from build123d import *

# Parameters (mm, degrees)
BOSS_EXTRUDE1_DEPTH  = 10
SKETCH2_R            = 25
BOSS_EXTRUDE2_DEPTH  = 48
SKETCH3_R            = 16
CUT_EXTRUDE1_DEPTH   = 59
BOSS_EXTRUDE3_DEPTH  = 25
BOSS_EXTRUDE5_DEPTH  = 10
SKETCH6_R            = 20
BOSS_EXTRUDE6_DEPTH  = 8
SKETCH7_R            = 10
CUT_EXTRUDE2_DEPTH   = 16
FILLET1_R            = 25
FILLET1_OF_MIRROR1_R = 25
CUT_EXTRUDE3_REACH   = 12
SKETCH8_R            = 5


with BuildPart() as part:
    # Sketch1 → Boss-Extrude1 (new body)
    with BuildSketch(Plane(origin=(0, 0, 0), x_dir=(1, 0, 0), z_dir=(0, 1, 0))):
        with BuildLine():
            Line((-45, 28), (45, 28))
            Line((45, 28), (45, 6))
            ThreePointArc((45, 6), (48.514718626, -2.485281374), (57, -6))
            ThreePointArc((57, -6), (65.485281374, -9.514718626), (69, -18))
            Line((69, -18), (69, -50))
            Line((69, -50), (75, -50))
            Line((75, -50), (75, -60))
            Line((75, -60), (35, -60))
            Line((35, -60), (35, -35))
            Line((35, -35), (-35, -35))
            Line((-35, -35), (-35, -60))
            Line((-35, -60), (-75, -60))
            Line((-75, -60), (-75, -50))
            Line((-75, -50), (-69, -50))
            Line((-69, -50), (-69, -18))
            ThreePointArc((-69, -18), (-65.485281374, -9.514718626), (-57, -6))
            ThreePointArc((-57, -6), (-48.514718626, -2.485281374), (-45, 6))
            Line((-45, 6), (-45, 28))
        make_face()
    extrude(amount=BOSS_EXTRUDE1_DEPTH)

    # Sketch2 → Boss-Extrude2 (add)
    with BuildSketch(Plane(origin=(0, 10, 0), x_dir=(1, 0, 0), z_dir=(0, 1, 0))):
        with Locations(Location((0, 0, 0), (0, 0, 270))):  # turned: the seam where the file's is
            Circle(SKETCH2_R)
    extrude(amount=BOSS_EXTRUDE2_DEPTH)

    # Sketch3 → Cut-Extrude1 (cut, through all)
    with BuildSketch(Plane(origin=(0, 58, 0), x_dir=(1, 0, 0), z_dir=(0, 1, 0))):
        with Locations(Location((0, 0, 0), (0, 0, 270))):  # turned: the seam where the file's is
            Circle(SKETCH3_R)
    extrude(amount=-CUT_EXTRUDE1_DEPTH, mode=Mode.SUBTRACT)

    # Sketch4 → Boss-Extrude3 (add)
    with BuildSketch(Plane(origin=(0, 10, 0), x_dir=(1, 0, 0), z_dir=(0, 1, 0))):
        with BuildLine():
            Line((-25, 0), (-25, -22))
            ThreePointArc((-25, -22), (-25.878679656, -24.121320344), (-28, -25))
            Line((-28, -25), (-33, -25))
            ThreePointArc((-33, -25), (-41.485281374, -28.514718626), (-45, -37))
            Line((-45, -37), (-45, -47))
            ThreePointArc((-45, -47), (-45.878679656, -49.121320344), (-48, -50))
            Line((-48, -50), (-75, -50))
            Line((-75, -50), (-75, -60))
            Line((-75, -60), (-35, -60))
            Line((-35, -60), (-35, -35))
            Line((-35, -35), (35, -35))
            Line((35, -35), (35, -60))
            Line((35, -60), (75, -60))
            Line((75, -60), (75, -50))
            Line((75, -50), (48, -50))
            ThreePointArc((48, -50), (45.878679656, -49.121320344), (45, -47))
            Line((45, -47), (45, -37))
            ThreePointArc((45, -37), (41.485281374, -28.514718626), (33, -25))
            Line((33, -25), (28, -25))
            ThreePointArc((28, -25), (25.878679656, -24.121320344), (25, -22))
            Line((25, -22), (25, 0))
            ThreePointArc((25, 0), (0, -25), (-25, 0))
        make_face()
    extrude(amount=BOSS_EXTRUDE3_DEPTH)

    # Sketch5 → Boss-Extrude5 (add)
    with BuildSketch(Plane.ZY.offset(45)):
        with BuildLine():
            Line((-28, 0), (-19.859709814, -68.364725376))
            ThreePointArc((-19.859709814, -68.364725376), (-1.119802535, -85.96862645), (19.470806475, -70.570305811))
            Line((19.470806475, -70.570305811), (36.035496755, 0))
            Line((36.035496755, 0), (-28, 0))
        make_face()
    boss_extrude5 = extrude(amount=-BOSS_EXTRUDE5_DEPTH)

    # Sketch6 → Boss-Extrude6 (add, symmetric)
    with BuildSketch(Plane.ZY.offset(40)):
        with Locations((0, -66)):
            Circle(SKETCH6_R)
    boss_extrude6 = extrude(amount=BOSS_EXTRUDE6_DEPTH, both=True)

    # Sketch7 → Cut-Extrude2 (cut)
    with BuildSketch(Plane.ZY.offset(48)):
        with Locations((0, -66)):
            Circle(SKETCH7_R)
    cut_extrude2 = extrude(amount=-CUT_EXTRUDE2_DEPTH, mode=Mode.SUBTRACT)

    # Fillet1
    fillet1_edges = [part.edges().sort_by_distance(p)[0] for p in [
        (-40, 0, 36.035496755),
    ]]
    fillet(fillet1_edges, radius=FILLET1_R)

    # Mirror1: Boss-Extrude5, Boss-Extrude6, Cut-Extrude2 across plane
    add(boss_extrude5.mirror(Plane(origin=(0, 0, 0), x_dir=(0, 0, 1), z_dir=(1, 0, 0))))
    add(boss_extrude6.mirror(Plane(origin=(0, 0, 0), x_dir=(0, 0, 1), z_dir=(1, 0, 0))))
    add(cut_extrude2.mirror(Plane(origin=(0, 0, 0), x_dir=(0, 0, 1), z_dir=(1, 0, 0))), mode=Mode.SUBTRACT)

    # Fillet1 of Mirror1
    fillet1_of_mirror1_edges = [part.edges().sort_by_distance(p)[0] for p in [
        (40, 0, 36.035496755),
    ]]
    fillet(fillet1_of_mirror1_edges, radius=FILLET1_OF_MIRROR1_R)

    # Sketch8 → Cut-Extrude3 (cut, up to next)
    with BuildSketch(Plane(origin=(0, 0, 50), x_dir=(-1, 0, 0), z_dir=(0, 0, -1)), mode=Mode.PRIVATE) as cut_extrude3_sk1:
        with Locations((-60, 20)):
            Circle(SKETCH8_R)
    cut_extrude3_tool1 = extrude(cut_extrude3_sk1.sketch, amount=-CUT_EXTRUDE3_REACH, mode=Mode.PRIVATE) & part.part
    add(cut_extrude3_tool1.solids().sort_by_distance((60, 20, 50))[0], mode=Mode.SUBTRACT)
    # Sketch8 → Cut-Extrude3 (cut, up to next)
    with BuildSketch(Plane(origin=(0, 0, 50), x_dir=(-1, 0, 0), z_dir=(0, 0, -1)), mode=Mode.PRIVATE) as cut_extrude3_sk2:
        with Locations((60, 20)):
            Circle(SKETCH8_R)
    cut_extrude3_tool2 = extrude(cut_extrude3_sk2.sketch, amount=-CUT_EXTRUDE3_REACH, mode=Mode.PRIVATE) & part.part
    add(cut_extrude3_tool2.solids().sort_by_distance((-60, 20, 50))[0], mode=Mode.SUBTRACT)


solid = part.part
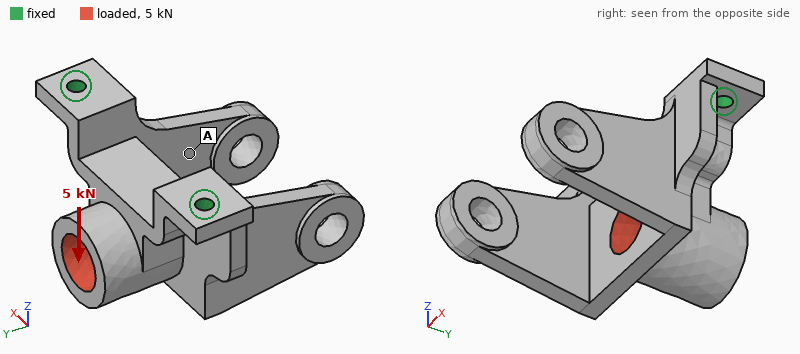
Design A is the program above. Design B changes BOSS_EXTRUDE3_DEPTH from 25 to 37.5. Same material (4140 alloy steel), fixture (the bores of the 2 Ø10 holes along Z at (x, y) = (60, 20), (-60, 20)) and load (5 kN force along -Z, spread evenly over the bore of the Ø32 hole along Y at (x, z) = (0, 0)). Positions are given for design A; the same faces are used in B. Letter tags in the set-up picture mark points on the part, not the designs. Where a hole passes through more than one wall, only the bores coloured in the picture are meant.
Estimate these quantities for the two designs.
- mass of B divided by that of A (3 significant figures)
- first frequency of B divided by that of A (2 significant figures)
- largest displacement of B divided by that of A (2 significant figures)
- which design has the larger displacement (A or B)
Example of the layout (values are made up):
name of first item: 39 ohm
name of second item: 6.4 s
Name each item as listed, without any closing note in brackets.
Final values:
mass of B divided by that of A: 1.10
first frequency of B divided by that of A: 1.1
largest displacement of B divided by that of A: 0.66
which design has the larger displacement: A
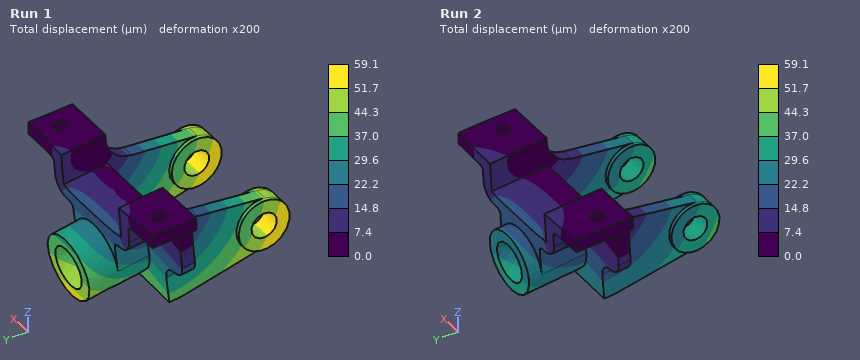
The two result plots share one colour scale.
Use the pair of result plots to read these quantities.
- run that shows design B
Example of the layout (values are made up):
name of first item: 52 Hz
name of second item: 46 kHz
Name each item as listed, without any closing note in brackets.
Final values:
run that shows design B: Run 2
